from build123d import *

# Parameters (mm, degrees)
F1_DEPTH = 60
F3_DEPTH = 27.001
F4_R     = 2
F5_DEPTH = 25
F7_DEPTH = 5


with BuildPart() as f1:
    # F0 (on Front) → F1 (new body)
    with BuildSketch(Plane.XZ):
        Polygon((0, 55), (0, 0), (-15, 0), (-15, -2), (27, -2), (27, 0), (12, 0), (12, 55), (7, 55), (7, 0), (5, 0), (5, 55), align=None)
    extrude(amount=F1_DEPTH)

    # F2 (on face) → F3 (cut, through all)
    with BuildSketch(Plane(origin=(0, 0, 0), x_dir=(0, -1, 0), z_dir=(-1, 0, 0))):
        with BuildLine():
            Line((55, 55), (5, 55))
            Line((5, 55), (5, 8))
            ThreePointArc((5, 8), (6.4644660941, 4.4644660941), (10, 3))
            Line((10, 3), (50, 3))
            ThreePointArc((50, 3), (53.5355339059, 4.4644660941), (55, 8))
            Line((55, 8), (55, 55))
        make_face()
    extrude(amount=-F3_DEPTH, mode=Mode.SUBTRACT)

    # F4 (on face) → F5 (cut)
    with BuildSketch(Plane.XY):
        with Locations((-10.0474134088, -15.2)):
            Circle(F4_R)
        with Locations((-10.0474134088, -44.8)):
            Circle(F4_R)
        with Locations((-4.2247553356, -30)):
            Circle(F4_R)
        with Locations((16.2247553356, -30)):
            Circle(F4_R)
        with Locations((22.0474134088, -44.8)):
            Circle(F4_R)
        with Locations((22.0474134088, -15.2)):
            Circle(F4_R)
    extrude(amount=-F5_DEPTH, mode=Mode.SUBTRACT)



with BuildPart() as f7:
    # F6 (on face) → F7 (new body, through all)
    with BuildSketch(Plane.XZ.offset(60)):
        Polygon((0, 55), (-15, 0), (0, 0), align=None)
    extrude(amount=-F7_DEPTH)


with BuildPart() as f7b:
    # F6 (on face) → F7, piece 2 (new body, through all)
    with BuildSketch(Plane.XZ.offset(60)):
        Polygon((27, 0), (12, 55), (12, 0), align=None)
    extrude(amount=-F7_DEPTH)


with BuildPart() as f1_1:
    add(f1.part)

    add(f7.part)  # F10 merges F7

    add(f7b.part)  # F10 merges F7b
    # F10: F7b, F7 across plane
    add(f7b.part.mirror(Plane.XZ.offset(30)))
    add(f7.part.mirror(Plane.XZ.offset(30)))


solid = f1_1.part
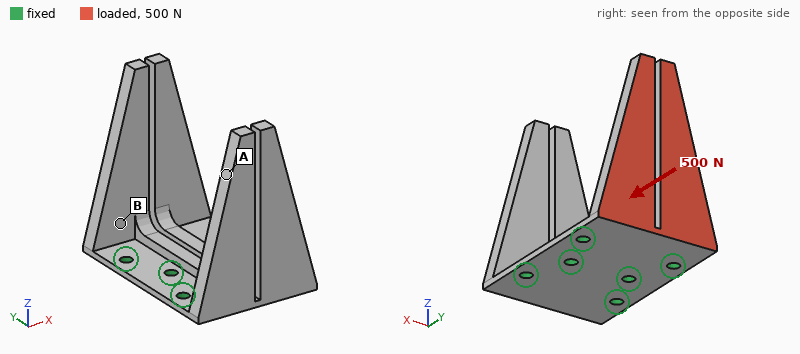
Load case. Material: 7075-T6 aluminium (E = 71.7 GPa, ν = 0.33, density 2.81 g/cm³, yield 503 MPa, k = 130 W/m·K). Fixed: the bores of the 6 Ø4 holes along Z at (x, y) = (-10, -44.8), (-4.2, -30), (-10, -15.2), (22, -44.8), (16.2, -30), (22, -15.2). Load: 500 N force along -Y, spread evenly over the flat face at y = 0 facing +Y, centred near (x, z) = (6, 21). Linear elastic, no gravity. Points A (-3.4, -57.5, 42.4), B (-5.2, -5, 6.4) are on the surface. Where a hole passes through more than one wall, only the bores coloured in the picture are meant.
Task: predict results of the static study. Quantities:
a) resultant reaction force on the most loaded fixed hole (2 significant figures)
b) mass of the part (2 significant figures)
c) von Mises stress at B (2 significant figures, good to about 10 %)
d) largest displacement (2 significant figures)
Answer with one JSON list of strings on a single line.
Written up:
["520 N", "57 g", "41 MPa", "1.1 mm"]
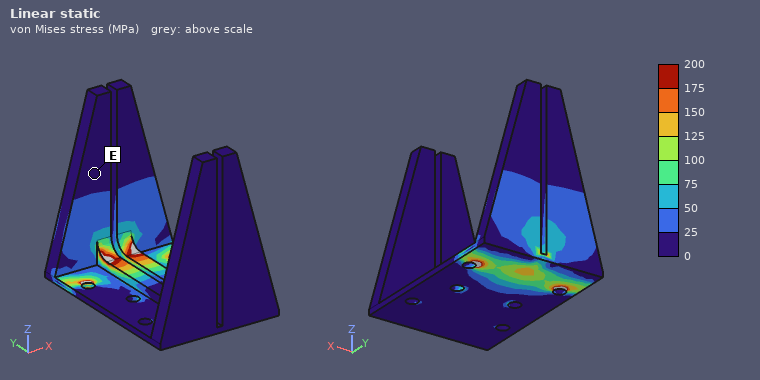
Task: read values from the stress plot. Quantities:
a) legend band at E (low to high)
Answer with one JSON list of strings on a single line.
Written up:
["0 to 25 MPa"]
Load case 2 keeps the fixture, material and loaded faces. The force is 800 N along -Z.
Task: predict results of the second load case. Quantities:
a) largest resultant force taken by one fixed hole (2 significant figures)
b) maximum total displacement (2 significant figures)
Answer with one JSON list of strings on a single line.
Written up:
["780 N", "0.87 mm"]
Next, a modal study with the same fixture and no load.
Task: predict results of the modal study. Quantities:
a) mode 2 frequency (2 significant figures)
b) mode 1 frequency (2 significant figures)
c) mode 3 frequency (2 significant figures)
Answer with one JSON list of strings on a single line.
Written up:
["970 Hz", "930 Hz", "1500 Hz"]
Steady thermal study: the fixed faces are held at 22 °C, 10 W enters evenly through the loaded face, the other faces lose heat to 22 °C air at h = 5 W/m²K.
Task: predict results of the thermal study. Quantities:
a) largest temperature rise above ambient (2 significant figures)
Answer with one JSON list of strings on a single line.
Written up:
["20 K"]
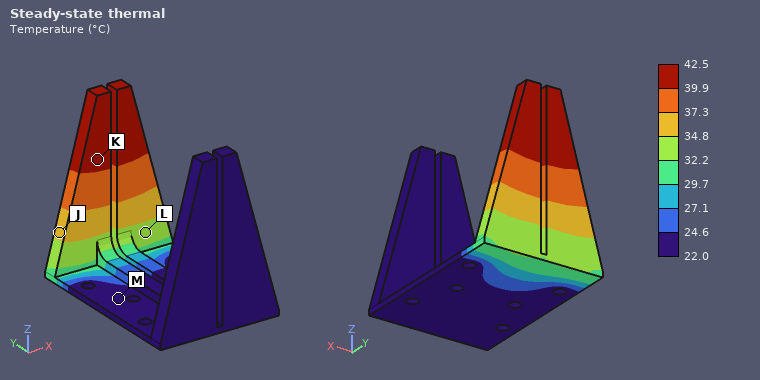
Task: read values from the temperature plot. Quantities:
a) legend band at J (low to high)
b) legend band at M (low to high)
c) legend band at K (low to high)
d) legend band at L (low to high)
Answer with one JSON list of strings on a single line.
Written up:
["34.8 to 37.3 °C", "22.0 to 24.6 °C", "39.9 to 42.5 °C", "32.2 to 34.8 °C"]
